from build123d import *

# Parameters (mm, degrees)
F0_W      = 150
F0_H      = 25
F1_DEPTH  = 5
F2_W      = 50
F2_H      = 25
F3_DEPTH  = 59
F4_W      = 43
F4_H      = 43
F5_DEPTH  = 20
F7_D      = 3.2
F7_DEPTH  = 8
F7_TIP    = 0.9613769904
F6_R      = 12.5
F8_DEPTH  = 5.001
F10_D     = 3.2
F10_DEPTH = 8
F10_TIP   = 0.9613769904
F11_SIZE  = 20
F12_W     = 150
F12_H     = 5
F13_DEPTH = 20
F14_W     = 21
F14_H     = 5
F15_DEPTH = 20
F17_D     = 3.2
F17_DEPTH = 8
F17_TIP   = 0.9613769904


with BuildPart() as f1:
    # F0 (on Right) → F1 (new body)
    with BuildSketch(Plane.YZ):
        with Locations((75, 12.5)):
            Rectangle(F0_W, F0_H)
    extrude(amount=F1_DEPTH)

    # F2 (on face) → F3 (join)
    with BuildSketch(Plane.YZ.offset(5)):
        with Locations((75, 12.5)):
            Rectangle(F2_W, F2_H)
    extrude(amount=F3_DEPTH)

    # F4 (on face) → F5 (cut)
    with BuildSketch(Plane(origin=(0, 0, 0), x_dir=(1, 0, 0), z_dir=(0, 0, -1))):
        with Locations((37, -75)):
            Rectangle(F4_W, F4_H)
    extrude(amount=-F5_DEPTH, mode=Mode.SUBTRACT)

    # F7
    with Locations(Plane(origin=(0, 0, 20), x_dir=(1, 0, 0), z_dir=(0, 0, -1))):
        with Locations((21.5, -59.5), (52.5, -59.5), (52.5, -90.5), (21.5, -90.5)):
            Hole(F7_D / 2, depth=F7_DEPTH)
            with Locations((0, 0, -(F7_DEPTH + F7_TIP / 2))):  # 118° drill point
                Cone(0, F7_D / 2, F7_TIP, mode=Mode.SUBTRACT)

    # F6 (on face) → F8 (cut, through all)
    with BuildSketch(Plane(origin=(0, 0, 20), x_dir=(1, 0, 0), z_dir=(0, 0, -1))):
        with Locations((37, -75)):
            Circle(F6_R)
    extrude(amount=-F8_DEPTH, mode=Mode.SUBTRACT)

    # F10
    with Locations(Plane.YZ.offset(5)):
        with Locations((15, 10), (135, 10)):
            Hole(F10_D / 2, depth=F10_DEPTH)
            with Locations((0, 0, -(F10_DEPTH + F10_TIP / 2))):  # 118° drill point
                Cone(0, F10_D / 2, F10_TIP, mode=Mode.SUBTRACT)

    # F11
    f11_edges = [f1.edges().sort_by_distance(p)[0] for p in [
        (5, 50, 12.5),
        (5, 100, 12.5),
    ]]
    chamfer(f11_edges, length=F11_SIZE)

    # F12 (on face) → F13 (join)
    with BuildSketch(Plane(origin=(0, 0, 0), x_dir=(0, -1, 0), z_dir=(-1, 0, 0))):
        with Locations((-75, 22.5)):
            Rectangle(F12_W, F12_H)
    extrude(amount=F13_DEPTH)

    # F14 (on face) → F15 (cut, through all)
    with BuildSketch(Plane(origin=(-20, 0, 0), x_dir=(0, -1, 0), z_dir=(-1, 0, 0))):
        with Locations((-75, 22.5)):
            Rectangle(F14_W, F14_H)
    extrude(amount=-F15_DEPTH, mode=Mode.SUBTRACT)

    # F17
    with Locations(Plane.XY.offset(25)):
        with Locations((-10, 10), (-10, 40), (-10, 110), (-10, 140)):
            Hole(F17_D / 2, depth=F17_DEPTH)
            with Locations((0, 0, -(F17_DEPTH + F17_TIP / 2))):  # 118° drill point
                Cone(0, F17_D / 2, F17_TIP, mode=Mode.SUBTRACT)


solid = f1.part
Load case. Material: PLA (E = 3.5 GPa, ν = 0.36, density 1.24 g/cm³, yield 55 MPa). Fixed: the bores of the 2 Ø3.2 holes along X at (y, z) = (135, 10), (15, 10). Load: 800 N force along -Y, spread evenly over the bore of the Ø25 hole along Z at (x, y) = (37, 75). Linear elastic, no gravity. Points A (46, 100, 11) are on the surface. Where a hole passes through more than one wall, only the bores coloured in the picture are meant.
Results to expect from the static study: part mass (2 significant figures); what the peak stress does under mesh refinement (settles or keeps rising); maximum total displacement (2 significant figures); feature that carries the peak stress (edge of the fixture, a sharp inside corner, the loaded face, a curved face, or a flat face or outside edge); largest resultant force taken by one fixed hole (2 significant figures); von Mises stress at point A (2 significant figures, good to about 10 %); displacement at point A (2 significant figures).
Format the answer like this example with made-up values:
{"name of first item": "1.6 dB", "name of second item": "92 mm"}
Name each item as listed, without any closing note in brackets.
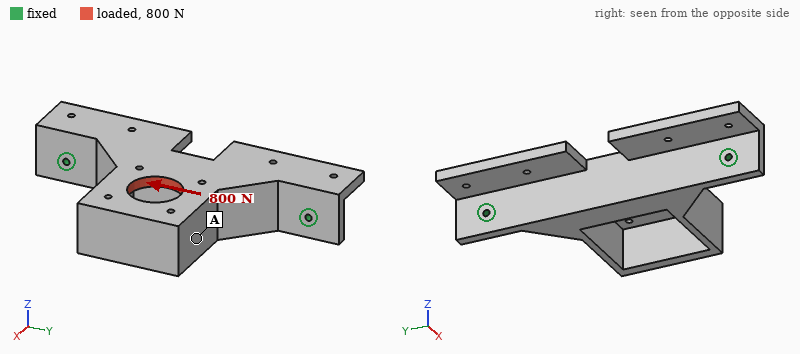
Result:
{"part mass": "94 g", "what the peak stress does under mesh refinement": "keeps rising", "maximum total displacement": "0.45 mm", "feature that carries the peak stress": "edge of the fixture", "largest resultant force taken by one fixed hole": "480 N", "von Mises stress at point A": "2.4 MPa", "displacement at point A": "0.31 mm"}
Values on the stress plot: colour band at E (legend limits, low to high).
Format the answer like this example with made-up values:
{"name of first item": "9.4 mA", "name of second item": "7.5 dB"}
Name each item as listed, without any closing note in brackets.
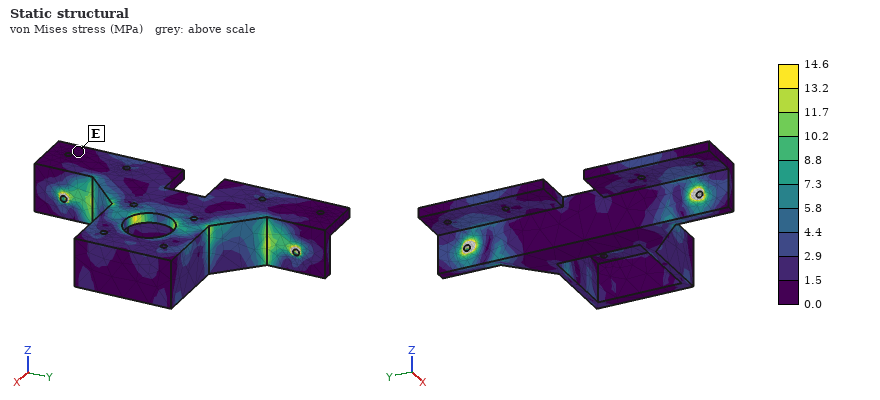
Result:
{"colour band at E": "0.0 to 1.5 MPa"}
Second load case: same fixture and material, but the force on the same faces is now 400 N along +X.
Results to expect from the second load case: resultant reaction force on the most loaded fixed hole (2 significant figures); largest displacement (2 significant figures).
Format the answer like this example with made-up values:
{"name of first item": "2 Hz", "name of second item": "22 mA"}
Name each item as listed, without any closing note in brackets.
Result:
{"resultant reaction force on the most loaded fixed hole": "250 N", "largest displacement": "1.4 mm"}
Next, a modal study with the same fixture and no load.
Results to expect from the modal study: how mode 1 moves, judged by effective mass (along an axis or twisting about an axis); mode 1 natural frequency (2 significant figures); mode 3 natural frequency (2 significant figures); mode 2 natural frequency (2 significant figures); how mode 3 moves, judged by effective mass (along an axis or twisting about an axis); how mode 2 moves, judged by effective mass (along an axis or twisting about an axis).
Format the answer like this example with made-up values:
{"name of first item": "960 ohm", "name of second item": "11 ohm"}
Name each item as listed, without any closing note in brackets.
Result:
{"how mode 1 moves, judged by effective mass": "along Z", "mode 1 natural frequency": "270 Hz", "mode 3 natural frequency": "980 Hz", "mode 2 natural frequency": "810 Hz", "how mode 3 moves, judged by effective mass": "along Y", "how mode 2 moves, judged by effective mass": "along X"}
